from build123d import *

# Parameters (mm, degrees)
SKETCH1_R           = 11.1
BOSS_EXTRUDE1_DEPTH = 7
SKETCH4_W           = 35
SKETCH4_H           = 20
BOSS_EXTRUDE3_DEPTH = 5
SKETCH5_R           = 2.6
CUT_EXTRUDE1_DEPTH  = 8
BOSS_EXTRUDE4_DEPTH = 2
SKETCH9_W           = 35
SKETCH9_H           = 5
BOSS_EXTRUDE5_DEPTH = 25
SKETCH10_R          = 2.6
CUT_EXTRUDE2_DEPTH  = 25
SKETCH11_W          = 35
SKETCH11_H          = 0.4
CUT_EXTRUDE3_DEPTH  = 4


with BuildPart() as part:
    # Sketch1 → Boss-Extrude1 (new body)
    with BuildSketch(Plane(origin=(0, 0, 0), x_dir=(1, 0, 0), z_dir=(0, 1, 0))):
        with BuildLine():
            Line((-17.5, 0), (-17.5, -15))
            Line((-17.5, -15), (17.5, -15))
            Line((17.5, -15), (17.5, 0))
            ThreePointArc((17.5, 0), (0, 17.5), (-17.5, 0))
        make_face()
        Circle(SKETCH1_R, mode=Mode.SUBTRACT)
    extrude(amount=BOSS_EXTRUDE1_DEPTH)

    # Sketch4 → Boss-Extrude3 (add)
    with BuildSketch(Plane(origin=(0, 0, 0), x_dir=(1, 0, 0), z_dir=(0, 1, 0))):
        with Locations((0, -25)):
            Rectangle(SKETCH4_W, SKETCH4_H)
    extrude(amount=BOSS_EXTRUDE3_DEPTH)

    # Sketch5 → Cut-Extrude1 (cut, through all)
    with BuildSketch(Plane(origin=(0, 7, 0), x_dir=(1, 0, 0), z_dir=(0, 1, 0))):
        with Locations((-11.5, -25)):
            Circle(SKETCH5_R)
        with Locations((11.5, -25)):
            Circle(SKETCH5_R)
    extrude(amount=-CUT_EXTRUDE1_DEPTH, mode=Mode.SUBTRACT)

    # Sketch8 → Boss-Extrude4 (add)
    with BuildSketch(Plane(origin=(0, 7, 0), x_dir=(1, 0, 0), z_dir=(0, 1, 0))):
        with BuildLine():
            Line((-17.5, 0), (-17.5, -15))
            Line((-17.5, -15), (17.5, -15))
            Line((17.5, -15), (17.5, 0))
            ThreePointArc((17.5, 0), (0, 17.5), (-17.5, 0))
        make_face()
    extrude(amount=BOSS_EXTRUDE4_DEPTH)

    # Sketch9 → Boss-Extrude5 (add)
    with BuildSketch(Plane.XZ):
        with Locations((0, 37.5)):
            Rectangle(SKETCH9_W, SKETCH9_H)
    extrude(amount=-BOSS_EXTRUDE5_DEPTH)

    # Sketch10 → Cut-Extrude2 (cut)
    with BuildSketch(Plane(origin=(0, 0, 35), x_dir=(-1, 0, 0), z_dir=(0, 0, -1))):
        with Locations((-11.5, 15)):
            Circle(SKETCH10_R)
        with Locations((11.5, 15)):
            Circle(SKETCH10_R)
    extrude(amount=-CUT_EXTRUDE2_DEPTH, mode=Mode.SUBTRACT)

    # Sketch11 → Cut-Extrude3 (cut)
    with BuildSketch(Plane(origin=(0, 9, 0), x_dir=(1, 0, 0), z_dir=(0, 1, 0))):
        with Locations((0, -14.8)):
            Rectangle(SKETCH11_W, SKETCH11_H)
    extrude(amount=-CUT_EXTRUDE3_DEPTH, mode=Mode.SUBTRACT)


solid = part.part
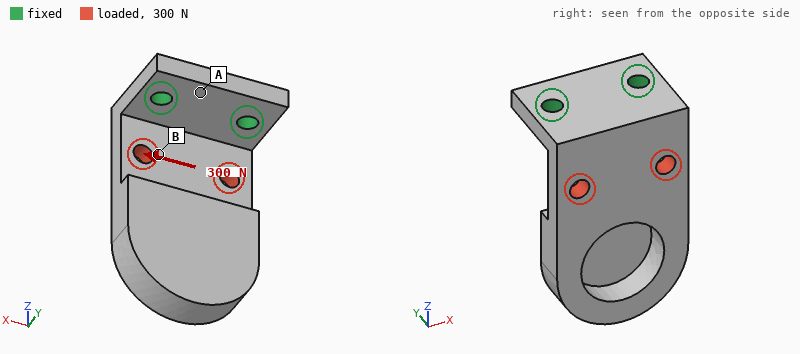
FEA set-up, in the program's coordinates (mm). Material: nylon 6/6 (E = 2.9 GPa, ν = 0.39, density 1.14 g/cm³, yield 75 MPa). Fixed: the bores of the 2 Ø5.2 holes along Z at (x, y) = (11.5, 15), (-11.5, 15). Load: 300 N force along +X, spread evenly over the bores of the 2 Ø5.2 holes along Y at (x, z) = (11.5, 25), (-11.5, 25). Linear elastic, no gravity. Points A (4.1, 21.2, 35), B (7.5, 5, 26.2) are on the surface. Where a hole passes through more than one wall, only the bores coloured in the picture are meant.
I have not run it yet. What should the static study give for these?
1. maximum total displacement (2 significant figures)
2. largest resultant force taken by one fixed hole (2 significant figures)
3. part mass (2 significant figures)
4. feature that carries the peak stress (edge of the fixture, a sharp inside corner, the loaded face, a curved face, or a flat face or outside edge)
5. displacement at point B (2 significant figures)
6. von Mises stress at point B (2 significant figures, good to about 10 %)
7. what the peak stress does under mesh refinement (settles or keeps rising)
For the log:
0.51 mm
250 N
16 g
edge of the fixture
0.15 mm
5.5 MPa
keeps rising
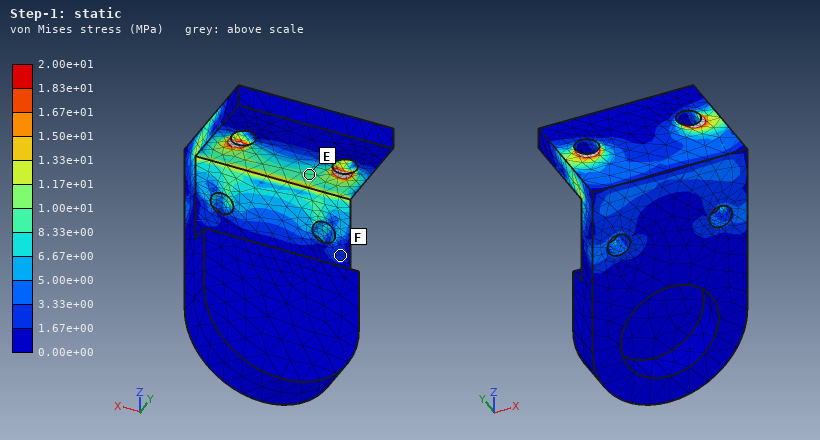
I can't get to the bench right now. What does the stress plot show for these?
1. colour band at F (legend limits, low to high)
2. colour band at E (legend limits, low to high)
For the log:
1.67e+00 to 3.33e+00 MPa
8.33e+00 to 1.00e+01 MPa
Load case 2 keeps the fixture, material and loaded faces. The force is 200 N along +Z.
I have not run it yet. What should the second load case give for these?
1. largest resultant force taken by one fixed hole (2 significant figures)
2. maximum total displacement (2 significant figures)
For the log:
100 N
0.71 mm
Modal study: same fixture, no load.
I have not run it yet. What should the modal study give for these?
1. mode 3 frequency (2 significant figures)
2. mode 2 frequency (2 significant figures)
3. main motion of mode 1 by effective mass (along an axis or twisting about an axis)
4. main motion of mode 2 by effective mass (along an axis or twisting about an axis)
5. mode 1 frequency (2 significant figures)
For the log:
1400 Hz
840 Hz
along Y
along X
330 Hz
